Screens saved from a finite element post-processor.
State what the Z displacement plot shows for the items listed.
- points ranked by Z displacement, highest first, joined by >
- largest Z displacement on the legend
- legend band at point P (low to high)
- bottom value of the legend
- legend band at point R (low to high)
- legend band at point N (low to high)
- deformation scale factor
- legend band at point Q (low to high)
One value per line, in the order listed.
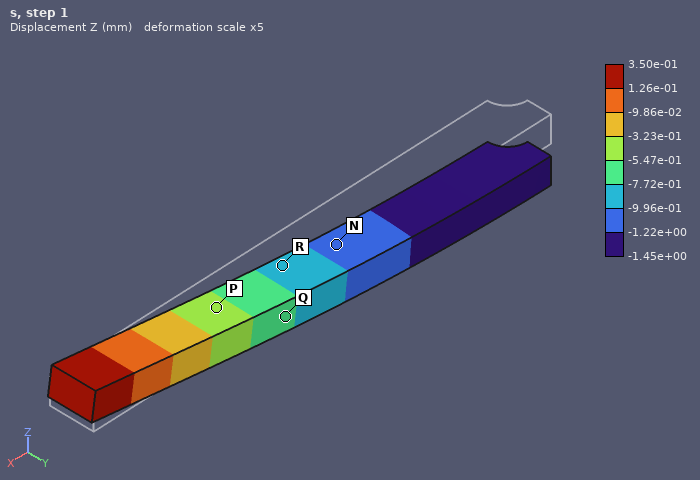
P > Q > R > N
3.50e-01 mm
-5.47e-01 to -3.23e-01 mm
-1.45e+00 mm
-9.96e-01 to -7.72e-01 mm
-1.22e+00 to -9.96e-01 mm
5
-7.72e-01 to -5.47e-01 mm
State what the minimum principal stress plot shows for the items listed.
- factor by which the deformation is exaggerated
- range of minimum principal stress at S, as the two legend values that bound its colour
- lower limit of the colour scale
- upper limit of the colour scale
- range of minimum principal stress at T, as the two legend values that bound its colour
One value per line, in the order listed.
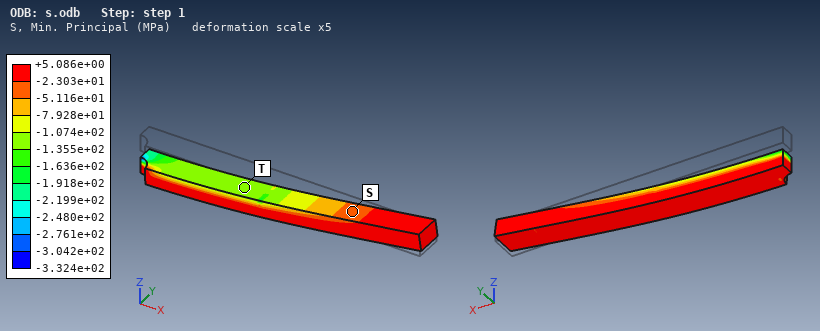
5
-5.116e+01 to -2.303e+01 MPa
-3.324e+02 MPa
+5.086e+00 MPa
-1.355e+02 to -1.074e+02 MPa
